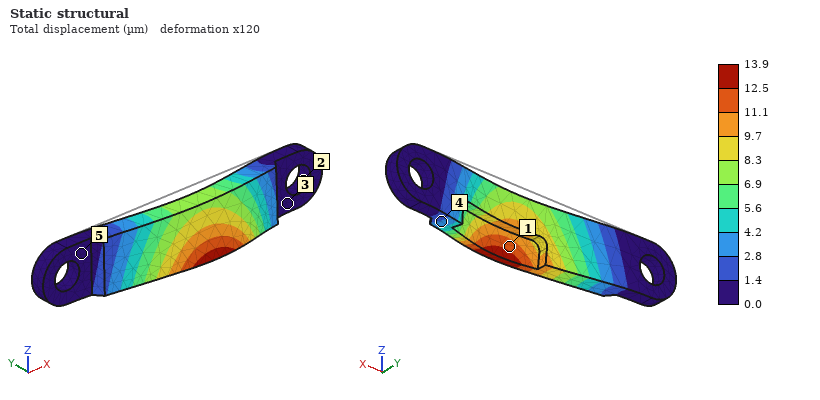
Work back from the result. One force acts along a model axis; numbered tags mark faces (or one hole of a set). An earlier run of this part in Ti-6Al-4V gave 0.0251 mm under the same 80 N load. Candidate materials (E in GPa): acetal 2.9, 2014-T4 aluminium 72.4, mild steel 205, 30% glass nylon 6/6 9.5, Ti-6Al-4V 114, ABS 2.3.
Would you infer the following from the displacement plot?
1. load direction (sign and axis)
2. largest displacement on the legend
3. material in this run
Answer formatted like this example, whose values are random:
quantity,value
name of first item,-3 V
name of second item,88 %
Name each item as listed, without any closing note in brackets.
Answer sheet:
quantity,value
load direction,-Y
largest displacement on the legend,13.9 µm
material in this run,mild steel
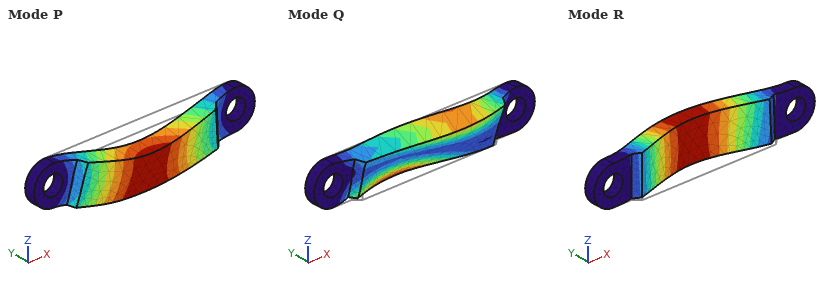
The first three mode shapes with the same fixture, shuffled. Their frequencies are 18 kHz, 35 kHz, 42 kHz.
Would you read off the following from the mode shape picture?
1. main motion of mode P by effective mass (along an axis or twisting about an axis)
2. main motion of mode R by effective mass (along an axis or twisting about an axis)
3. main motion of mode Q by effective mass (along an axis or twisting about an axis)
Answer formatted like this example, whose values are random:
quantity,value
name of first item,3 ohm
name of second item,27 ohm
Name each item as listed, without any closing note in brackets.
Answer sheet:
quantity,value
main motion of mode P by effective mass,along Z
main motion of mode R by effective mass,along Y
main motion of mode Q by effective mass,twisting about X
